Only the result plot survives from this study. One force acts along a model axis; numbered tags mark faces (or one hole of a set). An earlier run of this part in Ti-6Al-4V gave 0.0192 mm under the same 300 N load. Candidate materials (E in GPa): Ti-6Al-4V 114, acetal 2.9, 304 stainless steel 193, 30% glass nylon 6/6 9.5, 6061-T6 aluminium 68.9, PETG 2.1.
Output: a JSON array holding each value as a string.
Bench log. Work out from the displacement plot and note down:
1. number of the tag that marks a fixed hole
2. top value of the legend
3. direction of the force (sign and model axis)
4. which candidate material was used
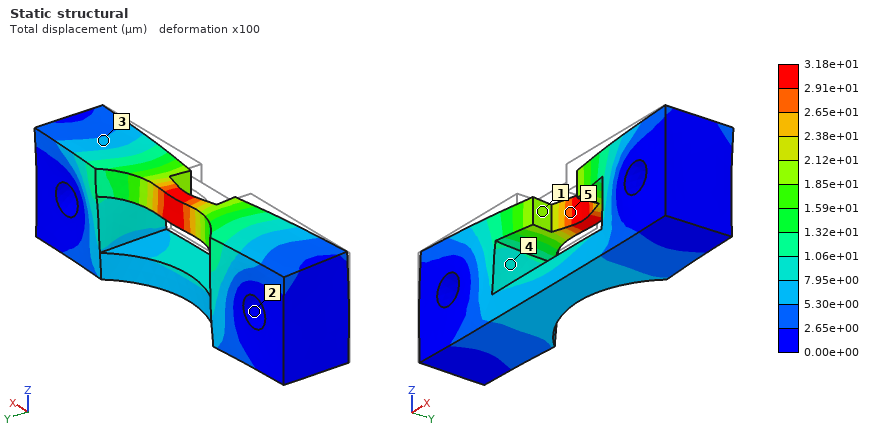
["2", "3.18e+01 µm", "+Y", "6061-T6 aluminium"]
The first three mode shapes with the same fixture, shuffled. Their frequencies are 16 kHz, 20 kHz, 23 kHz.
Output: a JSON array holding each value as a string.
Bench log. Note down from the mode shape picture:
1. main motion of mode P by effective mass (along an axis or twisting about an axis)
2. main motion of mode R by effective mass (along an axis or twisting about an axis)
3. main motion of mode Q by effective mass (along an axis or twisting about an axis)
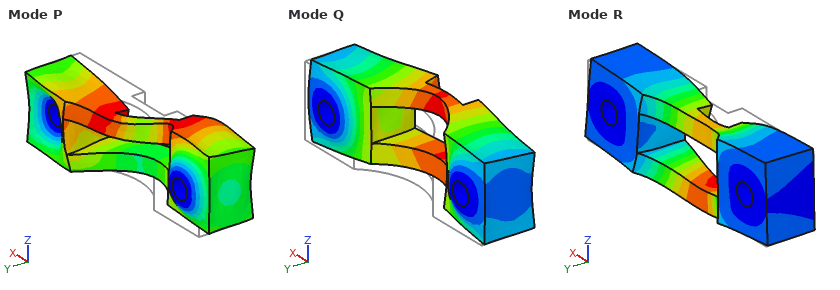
["twisting about Z", "along Z", "along Y"]
